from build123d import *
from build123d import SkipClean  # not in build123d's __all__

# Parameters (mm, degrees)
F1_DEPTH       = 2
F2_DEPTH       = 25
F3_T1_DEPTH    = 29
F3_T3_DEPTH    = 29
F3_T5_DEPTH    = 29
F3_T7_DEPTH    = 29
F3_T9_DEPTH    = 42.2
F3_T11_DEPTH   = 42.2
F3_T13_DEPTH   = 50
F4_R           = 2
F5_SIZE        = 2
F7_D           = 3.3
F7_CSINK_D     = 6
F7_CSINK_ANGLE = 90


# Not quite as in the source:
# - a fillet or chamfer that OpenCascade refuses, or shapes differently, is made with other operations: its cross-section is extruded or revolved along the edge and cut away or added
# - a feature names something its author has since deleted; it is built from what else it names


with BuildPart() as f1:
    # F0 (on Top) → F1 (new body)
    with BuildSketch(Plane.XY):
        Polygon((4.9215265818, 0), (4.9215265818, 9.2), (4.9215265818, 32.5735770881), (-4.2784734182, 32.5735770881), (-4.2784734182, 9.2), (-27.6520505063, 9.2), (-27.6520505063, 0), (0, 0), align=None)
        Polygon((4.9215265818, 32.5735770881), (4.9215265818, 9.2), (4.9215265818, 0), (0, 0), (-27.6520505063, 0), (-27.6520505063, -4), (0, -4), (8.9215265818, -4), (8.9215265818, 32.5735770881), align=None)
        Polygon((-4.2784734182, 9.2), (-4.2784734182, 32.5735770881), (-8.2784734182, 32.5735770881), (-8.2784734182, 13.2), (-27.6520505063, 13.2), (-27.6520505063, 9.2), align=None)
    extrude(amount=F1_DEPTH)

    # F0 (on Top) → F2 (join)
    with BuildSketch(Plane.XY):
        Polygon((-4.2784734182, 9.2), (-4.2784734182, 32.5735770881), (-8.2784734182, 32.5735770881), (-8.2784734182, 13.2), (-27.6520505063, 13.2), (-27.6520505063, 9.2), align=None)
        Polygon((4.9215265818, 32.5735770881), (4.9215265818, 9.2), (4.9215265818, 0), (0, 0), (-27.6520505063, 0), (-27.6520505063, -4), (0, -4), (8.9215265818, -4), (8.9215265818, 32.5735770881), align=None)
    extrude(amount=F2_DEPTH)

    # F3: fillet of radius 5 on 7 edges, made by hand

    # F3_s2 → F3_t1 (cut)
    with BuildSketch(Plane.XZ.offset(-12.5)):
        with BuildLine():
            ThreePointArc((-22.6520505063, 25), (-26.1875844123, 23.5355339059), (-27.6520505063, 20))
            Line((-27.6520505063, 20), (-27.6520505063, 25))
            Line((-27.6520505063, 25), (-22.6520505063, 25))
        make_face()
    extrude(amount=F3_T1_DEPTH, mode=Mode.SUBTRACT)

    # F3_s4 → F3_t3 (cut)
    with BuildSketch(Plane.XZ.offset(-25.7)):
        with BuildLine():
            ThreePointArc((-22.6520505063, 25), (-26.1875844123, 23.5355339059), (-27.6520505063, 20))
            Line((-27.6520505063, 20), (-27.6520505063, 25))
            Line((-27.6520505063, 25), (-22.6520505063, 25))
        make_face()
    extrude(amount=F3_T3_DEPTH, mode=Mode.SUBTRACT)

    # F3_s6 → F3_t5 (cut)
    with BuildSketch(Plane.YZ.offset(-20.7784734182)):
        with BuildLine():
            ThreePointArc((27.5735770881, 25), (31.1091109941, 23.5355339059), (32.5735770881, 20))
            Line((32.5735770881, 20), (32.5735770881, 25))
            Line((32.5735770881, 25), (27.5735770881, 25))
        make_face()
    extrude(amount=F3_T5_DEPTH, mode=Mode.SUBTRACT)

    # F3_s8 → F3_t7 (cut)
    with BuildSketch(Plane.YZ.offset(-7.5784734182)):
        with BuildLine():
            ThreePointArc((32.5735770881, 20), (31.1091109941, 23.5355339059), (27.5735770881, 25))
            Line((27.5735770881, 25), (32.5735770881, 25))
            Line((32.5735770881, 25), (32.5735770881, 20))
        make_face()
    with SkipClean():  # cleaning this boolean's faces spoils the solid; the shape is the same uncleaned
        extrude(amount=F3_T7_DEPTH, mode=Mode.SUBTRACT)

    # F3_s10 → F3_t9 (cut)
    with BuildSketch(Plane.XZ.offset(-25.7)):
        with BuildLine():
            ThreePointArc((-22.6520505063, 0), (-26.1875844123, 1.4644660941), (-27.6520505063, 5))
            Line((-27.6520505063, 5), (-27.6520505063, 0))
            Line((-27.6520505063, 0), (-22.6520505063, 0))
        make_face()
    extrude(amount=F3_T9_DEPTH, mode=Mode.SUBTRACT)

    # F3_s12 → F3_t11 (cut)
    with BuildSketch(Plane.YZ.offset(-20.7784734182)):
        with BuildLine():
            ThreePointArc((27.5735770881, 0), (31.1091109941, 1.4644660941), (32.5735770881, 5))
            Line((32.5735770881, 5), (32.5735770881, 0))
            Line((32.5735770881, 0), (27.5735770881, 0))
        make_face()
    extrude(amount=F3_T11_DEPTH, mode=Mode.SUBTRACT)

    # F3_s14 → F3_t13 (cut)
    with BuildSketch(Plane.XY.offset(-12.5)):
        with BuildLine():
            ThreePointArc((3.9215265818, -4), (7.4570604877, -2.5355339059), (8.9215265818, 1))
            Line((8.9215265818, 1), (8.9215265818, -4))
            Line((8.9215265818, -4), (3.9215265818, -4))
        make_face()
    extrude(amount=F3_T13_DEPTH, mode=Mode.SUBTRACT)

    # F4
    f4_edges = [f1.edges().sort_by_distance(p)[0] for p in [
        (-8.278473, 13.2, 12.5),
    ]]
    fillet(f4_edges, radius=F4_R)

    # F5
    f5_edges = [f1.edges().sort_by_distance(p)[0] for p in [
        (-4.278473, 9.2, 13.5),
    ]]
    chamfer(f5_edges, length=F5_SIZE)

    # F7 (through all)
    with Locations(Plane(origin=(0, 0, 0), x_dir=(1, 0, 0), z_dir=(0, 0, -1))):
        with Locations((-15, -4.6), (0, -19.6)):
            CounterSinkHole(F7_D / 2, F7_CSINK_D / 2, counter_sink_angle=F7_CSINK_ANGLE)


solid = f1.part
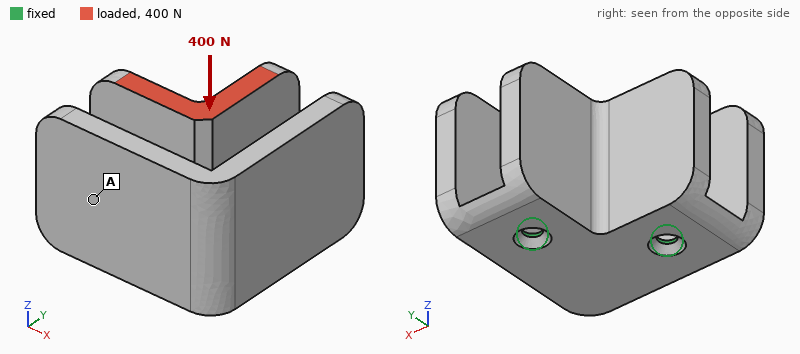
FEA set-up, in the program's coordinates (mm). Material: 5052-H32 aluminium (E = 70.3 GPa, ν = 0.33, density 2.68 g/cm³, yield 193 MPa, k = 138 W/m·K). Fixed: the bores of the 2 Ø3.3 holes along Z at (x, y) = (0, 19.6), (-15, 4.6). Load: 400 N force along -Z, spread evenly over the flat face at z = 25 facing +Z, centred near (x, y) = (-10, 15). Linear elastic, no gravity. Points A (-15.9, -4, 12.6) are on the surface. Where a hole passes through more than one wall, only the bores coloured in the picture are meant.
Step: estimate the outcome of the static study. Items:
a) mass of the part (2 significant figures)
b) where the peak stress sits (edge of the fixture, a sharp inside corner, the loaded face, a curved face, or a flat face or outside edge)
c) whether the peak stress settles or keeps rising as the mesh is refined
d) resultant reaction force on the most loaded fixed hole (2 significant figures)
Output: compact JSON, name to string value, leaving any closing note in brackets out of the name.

{"mass of the part": "31 g", "where the peak stress sits": "edge of the fixture", "whether the peak stress settles or keeps rising as the mesh is refined": "keeps rising", "resultant reaction force on the most loaded fixed hole": "210 N"}
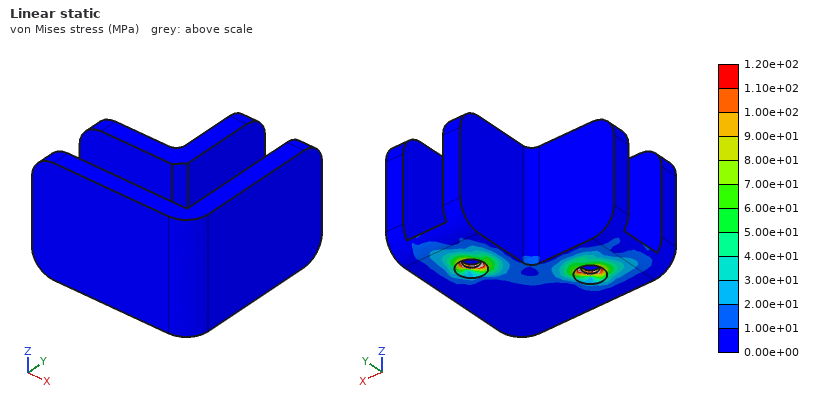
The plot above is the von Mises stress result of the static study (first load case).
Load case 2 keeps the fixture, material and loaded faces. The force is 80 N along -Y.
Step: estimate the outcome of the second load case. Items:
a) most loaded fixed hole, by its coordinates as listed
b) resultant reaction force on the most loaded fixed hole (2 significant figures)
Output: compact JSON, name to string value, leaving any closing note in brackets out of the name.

{"most loaded fixed hole, by its coordinates as listed": "(0, 19.6)", "resultant reaction force on the most loaded fixed hole": "100 N"}
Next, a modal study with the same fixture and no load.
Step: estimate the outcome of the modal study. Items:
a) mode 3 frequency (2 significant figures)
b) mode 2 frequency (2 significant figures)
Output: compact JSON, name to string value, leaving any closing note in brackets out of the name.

{"mode 3 frequency": "2900 Hz", "mode 2 frequency": "2800 Hz"}
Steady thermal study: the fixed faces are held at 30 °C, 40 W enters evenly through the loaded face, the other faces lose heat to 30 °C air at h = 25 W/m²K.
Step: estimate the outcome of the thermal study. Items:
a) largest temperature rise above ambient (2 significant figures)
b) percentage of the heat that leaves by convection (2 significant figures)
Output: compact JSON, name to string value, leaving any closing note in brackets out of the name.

{"largest temperature rise above ambient": "74 K", "percentage of the heat that leaves by convection": "12 %"}
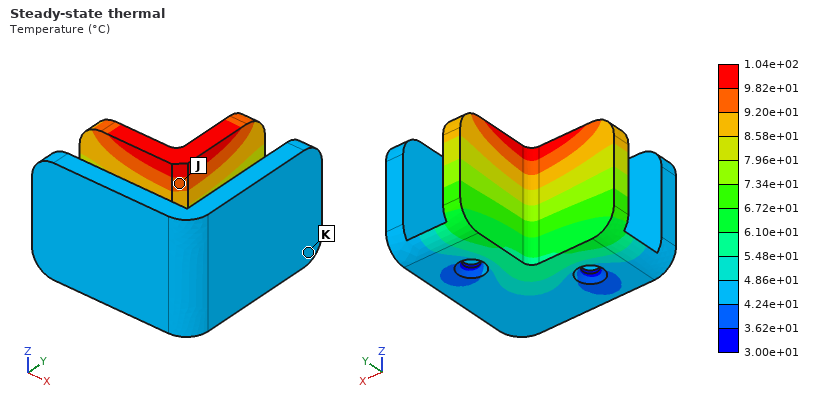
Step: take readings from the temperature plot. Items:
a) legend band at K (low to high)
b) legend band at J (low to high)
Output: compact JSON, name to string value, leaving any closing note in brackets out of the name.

{"legend band at K": "4.24e+01 to 4.86e+01 °C", "legend band at J": "9.20e+01 to 9.82e+01 °C"}
